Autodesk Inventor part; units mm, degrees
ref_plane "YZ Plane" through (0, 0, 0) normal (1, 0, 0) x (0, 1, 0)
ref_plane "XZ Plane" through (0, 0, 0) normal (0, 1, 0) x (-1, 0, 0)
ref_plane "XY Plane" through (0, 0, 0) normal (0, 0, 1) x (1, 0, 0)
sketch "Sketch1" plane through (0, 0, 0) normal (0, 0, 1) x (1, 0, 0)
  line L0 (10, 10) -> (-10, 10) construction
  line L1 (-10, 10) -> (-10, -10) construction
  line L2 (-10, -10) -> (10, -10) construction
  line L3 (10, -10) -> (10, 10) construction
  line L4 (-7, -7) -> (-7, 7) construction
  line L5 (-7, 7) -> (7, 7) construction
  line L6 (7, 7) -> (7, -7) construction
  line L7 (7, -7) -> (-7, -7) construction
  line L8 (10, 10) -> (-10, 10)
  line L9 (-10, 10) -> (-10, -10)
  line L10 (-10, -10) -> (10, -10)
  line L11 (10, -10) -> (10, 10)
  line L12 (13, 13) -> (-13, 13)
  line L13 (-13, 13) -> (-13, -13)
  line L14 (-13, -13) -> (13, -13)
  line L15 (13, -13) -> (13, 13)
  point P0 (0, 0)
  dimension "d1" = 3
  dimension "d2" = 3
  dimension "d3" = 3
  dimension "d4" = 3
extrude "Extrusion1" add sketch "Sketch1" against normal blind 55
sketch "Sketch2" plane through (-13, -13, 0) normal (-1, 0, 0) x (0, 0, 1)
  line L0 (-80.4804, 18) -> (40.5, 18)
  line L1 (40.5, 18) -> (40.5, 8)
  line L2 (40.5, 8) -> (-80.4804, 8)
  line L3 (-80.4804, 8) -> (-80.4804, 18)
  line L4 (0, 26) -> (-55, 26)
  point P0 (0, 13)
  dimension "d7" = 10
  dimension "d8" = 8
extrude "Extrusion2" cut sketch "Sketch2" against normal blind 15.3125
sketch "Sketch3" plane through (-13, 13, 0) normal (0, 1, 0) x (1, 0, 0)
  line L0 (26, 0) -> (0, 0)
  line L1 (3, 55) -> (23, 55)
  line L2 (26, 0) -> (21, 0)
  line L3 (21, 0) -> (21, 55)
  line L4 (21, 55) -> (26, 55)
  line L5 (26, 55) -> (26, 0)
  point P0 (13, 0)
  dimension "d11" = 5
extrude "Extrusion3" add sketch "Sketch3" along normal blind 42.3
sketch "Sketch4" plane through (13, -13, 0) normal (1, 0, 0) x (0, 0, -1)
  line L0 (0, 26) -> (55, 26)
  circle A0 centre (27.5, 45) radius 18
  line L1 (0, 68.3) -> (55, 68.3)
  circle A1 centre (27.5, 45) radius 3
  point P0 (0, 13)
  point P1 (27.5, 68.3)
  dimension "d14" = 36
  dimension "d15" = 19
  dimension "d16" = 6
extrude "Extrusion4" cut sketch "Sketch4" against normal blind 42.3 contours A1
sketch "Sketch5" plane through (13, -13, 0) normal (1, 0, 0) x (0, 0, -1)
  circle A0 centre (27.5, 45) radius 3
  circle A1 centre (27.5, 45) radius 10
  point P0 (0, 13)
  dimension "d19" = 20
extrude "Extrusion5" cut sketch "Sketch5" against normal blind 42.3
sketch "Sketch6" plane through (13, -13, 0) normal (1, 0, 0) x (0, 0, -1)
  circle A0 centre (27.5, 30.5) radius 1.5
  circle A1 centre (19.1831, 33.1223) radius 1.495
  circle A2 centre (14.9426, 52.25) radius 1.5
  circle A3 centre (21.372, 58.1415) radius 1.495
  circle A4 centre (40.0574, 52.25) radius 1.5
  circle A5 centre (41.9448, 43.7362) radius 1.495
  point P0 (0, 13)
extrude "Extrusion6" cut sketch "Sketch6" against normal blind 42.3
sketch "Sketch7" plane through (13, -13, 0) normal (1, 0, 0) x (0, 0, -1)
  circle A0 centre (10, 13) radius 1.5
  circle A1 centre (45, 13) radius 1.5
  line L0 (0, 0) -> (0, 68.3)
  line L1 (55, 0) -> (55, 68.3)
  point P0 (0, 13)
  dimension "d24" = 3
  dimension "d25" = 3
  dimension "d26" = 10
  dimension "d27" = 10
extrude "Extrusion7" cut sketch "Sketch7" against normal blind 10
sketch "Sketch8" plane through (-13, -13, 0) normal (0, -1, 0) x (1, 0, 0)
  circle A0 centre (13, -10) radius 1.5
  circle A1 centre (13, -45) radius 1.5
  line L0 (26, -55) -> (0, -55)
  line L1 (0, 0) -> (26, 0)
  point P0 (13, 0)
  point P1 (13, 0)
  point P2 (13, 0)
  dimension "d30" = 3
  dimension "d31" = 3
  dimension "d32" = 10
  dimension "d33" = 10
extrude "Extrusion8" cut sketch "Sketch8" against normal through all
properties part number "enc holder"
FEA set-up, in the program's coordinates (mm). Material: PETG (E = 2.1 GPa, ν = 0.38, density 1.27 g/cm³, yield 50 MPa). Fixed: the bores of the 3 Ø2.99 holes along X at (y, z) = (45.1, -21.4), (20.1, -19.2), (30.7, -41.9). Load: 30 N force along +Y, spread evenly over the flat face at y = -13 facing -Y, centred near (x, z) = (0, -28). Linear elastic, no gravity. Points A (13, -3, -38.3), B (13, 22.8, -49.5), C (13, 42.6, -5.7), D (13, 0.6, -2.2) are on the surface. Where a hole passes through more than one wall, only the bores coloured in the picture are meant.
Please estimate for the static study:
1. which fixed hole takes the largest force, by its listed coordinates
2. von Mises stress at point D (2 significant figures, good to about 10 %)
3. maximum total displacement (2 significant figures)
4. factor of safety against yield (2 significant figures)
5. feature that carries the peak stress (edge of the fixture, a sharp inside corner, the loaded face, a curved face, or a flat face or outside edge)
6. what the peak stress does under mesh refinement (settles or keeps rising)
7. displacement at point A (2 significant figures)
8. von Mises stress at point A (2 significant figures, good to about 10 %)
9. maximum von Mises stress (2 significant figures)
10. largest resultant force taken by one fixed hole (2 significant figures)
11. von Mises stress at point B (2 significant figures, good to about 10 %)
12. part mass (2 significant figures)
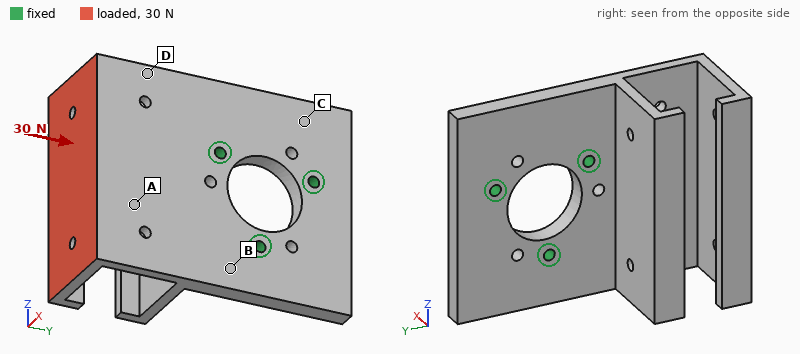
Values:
(20.1, -19.2)
4.3 MPa
1.0 mm
5.6
a curved face
settles
0.21 mm
3.6 MPa
9.0 MPa
16 N
0.89 MPa
30 g
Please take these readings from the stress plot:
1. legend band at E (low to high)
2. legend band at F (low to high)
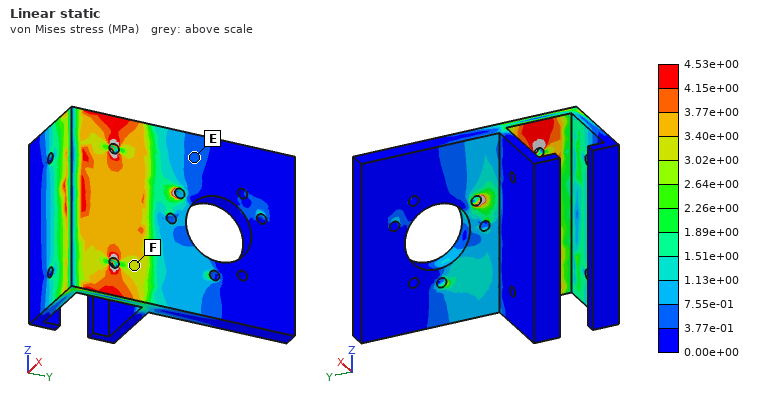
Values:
3.77e-01 to 7.55e-01 MPa
3.02e+00 to 3.40e+00 MPa
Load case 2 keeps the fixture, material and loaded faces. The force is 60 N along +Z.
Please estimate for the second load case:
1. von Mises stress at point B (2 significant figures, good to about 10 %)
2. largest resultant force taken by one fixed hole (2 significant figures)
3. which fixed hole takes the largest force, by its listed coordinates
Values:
3.1 MPa
84 N
(20.1, -19.2)
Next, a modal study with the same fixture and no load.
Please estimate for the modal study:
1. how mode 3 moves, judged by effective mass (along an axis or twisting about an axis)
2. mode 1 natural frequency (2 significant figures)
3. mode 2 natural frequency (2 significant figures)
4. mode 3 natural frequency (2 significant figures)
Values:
along X
280 Hz
440 Hz
640 Hz
